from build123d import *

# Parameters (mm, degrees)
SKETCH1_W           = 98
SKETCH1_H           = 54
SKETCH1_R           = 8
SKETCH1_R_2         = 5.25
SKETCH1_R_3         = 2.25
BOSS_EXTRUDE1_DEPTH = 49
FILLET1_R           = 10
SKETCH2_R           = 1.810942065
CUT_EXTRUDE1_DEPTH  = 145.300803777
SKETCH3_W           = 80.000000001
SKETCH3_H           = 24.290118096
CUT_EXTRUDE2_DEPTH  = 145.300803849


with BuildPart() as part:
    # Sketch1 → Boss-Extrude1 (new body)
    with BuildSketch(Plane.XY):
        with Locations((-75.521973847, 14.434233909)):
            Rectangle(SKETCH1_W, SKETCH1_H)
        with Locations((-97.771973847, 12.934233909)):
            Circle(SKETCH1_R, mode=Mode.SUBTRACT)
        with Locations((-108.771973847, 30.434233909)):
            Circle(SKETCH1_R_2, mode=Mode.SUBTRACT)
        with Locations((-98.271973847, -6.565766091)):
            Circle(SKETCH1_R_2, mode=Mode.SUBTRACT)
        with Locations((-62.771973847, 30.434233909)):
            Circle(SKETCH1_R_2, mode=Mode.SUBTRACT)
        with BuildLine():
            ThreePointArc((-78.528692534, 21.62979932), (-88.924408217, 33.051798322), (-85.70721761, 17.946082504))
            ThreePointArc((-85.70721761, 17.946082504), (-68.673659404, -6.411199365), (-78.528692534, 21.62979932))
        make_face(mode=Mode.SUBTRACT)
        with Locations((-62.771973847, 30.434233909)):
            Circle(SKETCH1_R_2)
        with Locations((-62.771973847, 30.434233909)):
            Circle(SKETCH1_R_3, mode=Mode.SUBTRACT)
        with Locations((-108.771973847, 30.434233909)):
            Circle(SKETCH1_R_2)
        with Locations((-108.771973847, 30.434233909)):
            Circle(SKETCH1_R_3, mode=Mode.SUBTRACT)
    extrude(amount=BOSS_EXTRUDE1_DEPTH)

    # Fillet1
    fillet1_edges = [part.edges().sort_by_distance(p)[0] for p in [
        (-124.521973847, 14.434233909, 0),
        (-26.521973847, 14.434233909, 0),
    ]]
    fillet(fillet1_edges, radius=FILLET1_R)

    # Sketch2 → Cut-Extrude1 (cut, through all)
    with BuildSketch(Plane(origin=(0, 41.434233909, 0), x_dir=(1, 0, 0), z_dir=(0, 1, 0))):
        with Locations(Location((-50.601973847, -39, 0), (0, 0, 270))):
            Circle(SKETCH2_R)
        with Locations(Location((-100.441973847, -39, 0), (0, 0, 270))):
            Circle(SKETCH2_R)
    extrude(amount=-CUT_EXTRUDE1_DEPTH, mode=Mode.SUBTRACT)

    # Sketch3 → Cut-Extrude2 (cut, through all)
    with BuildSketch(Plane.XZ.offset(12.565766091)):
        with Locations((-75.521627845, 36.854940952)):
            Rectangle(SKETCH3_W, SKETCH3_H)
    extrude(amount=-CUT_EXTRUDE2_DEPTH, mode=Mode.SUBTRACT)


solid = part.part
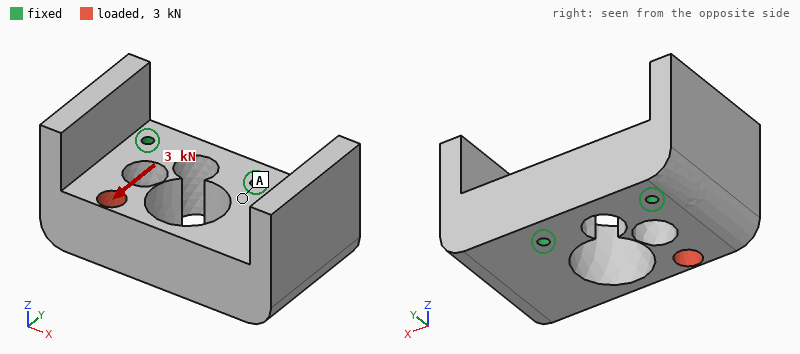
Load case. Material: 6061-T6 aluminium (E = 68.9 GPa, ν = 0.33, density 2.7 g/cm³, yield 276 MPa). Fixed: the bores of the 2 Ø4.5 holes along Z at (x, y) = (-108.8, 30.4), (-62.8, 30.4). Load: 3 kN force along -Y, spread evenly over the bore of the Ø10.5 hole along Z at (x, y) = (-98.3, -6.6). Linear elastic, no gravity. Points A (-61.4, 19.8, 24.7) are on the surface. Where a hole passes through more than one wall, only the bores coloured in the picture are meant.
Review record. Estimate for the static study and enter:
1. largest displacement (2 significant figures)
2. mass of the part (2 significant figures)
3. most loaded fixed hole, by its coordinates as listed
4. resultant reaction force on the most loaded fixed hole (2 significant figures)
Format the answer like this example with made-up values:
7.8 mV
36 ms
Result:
19 µm
330 g
(-108.8, 30.4)
2.5 kN
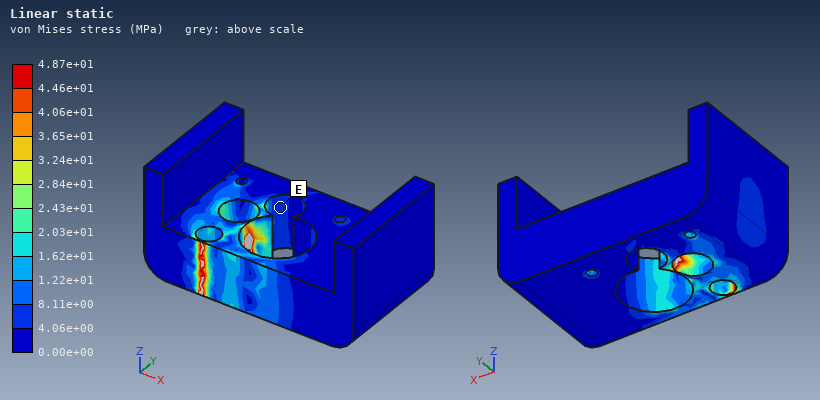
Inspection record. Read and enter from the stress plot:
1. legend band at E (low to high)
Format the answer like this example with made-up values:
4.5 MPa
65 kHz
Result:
4.06e+00 to 8.11e+00 MPa
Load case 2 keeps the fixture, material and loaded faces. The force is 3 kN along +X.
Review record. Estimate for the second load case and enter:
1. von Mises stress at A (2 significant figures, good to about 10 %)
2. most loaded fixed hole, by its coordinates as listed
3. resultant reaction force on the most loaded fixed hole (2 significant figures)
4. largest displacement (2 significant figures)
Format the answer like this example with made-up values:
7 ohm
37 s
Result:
8.7 MPa
(-108.8, 30.4)
2.6 kN
37 µm
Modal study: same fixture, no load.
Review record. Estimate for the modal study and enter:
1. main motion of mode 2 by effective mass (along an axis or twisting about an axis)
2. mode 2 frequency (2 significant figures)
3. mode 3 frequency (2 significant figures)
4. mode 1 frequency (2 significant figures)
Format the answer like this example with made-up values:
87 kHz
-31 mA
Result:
along Z
4300 Hz
5600 Hz
3900 Hz
